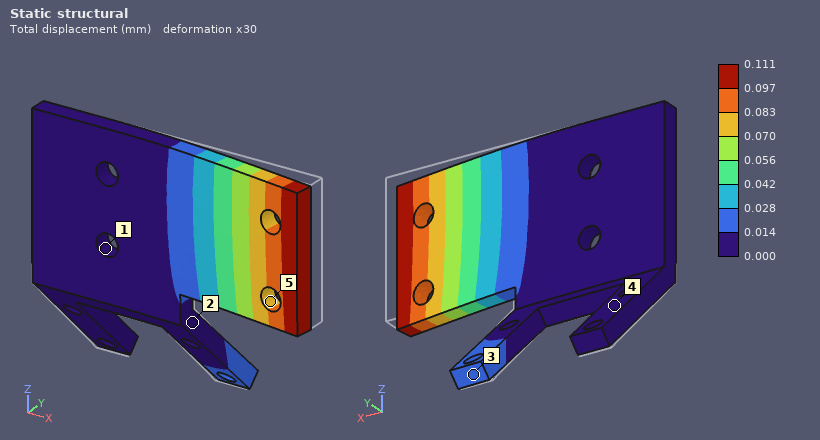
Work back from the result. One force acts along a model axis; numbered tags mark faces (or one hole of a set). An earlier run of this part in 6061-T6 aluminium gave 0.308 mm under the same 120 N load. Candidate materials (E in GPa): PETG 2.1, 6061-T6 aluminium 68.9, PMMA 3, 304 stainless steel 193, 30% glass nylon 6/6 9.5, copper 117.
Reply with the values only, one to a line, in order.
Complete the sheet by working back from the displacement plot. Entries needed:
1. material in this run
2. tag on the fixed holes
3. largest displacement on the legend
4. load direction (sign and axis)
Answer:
304 stainless steel
1
0.111 mm
-Y
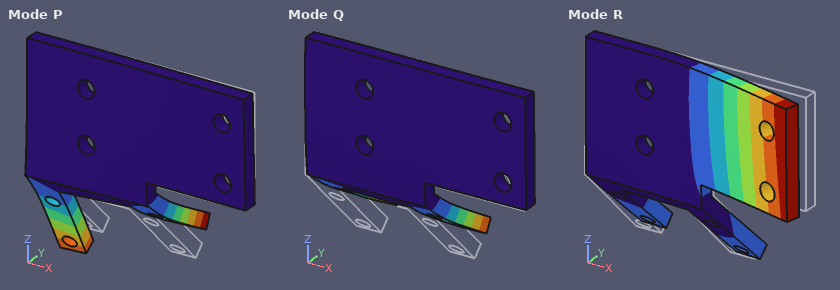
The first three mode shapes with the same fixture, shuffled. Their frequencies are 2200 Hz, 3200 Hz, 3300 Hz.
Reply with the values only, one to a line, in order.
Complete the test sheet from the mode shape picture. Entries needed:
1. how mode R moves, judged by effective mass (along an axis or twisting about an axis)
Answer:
along Y
